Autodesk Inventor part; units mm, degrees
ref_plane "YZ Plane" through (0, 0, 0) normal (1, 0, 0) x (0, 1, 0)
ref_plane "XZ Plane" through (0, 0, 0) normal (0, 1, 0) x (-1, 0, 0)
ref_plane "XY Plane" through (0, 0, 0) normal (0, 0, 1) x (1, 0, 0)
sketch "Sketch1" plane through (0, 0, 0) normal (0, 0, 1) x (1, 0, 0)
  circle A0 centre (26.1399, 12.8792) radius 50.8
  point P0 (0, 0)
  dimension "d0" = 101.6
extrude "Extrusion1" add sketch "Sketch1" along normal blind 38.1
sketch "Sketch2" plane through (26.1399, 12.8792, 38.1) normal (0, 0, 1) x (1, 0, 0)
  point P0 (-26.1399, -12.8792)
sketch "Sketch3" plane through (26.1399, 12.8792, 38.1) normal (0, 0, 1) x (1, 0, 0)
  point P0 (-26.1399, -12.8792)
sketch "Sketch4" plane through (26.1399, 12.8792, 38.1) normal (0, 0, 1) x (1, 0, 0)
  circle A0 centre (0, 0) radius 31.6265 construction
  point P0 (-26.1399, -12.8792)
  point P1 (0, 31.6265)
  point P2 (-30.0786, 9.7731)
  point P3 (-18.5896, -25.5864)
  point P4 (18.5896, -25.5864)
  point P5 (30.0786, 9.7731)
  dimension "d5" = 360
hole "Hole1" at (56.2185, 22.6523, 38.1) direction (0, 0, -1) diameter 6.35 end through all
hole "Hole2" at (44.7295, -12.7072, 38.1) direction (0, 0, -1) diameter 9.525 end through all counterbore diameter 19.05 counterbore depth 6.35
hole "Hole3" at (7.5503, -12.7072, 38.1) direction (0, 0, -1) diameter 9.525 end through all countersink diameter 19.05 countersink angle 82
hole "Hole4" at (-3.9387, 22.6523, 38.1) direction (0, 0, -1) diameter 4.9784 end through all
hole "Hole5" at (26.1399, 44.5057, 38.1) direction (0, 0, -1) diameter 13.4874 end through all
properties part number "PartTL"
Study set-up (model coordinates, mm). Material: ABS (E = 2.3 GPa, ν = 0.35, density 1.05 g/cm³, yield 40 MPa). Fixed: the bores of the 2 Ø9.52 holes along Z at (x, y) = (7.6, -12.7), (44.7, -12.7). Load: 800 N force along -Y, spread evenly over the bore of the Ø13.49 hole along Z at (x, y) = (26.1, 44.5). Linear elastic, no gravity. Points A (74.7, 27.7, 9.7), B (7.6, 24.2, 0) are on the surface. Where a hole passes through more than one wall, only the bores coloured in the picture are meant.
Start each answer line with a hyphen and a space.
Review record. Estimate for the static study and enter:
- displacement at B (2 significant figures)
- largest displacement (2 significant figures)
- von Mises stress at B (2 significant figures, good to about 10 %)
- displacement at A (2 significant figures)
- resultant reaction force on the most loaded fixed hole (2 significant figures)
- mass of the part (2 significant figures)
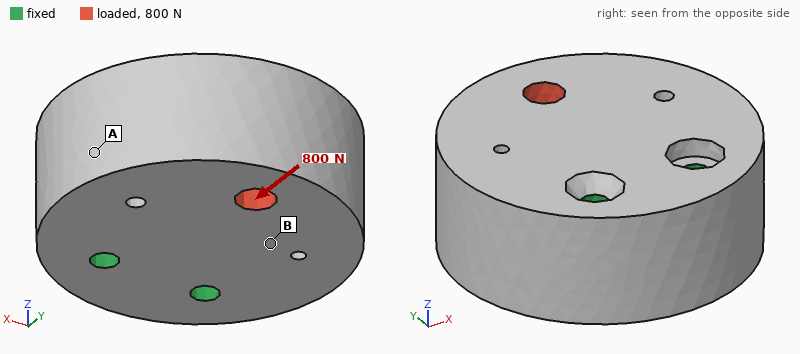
- 4.9 µm
- 16 µm
- 0.34 MPa
- 4.8 µm
- 410 N
- 310 g
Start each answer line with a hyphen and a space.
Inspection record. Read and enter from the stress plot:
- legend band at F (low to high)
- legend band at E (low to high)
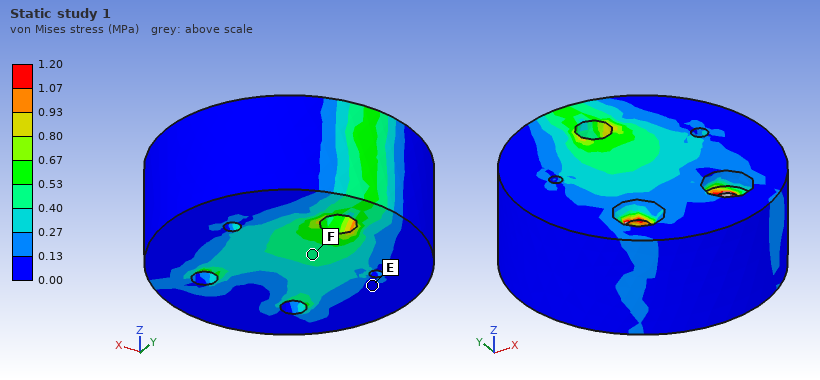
- 0.40 to 0.53 MPa
- 0.00 to 0.13 MPa
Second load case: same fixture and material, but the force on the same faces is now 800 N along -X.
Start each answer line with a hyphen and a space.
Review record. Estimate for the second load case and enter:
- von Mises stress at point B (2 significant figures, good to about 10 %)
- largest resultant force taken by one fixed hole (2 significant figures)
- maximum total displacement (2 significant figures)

- 0.58 MPa
- 1.1 kN
- 59 µm
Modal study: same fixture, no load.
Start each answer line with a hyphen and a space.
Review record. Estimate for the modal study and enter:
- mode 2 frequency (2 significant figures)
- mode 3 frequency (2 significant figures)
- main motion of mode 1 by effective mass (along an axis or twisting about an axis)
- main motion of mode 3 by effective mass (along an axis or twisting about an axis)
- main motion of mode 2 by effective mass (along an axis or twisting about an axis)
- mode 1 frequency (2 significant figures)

- 1700 Hz
- 2300 Hz
- along Z
- twisting about Y
- along X
- 1300 Hz
